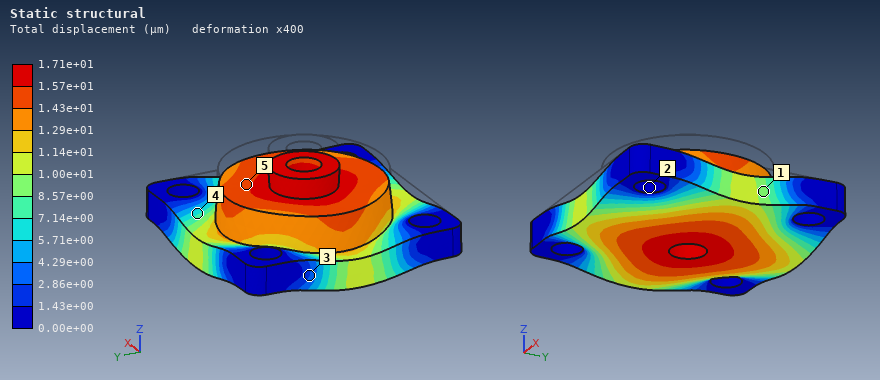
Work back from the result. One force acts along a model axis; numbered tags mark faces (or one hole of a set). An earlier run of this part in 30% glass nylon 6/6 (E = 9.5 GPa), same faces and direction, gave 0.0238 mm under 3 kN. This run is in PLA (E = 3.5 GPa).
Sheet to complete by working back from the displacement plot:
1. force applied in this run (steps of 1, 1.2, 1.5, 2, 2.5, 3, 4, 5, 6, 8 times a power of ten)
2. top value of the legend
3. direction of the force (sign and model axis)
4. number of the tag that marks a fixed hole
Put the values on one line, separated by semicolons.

800 N; 1.71e+01 µm; -Z; 2
